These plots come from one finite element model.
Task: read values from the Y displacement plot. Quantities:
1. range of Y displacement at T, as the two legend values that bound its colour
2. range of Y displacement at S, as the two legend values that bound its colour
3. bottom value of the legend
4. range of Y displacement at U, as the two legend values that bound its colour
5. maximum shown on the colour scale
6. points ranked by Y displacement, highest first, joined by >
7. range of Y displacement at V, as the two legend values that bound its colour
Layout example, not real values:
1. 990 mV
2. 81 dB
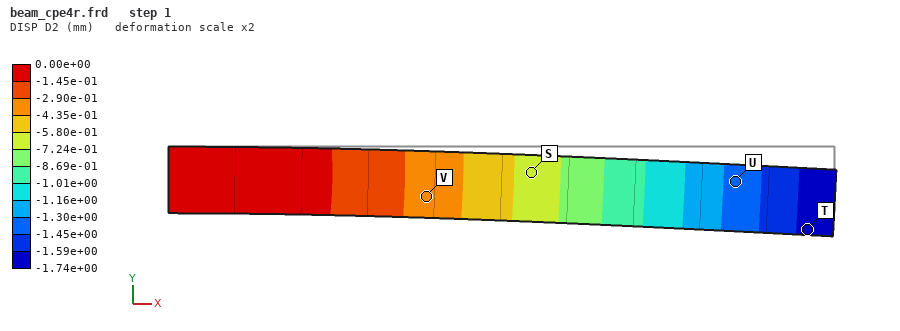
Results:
1. -1.74e+00 to -1.59e+00 mm
2. -7.24e-01 to -5.80e-01 mm
3. -1.74e+00 mm
4. -1.45e+00 to -1.30e+00 mm
5. 0.00e+00 mm
6. V > S > U > T
7. -4.35e-01 to -2.90e-01 mm
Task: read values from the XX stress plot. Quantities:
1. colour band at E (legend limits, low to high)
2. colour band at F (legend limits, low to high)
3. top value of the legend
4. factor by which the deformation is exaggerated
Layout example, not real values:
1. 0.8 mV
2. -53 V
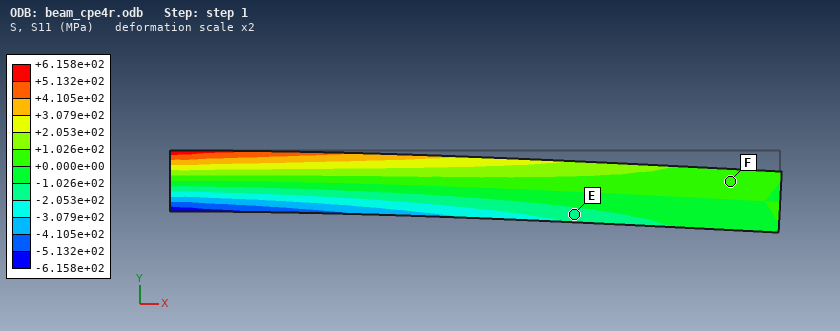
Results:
1. -2.053e+02 to -1.026e+02 MPa
2. +0.000e+00 to +1.026e+02 MPa
3. +6.158e+02 MPa
4. 2
